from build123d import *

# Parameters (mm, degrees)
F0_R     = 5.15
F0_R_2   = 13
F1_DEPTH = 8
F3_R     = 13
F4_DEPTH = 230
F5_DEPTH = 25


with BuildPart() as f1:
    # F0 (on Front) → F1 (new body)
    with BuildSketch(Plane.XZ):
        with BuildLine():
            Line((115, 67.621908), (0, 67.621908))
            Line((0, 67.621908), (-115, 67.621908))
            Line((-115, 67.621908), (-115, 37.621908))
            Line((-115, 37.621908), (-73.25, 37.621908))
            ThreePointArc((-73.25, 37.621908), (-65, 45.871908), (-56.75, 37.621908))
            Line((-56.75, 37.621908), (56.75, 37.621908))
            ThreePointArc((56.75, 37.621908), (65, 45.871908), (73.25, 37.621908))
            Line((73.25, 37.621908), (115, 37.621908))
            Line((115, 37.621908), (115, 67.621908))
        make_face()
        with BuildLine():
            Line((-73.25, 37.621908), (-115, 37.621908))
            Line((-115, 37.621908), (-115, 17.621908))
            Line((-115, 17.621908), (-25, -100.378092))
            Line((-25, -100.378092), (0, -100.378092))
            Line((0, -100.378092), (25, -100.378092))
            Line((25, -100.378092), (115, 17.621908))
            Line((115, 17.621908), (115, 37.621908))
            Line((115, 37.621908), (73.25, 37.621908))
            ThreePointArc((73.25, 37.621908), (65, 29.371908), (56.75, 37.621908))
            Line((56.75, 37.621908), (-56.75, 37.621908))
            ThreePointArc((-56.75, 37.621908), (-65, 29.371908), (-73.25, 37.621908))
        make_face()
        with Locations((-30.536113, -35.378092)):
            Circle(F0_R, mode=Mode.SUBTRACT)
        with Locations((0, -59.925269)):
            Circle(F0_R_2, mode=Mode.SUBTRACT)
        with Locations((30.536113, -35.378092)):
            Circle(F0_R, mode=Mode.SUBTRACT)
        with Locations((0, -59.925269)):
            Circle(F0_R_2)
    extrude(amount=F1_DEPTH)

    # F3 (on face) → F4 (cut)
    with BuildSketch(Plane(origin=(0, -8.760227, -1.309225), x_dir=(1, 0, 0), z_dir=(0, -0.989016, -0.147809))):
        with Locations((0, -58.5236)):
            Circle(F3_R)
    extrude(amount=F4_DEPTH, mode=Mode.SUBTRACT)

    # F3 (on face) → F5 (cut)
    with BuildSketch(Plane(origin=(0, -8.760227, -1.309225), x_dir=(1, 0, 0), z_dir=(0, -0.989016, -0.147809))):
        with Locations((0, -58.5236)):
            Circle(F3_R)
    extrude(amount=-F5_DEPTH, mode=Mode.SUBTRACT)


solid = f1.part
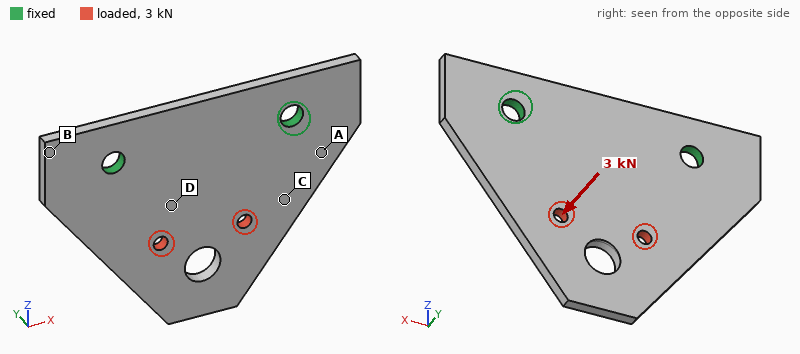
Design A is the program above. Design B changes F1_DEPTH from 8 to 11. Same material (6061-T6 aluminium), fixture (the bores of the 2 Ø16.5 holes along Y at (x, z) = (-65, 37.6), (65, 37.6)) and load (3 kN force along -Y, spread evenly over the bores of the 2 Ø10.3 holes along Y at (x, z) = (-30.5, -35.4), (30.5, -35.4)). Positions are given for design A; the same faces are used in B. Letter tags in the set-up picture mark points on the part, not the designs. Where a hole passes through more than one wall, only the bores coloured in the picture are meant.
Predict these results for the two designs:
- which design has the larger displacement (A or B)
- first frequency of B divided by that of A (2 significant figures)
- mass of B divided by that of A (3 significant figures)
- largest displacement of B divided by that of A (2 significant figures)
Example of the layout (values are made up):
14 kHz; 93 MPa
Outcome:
A; 1.3; 1.38; 0.40
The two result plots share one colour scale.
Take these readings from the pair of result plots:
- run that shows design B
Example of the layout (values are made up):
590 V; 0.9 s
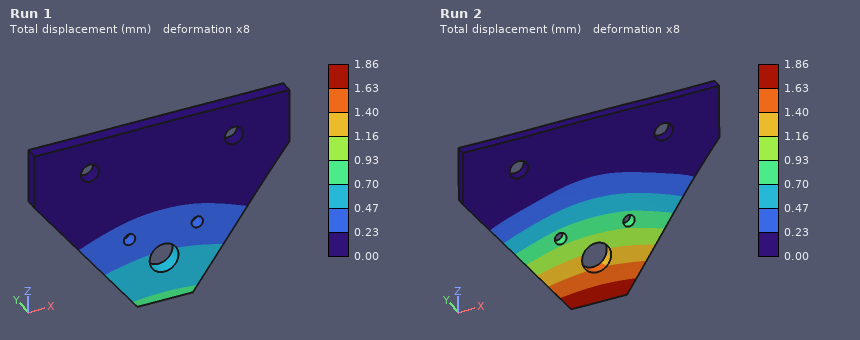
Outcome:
Run 1
